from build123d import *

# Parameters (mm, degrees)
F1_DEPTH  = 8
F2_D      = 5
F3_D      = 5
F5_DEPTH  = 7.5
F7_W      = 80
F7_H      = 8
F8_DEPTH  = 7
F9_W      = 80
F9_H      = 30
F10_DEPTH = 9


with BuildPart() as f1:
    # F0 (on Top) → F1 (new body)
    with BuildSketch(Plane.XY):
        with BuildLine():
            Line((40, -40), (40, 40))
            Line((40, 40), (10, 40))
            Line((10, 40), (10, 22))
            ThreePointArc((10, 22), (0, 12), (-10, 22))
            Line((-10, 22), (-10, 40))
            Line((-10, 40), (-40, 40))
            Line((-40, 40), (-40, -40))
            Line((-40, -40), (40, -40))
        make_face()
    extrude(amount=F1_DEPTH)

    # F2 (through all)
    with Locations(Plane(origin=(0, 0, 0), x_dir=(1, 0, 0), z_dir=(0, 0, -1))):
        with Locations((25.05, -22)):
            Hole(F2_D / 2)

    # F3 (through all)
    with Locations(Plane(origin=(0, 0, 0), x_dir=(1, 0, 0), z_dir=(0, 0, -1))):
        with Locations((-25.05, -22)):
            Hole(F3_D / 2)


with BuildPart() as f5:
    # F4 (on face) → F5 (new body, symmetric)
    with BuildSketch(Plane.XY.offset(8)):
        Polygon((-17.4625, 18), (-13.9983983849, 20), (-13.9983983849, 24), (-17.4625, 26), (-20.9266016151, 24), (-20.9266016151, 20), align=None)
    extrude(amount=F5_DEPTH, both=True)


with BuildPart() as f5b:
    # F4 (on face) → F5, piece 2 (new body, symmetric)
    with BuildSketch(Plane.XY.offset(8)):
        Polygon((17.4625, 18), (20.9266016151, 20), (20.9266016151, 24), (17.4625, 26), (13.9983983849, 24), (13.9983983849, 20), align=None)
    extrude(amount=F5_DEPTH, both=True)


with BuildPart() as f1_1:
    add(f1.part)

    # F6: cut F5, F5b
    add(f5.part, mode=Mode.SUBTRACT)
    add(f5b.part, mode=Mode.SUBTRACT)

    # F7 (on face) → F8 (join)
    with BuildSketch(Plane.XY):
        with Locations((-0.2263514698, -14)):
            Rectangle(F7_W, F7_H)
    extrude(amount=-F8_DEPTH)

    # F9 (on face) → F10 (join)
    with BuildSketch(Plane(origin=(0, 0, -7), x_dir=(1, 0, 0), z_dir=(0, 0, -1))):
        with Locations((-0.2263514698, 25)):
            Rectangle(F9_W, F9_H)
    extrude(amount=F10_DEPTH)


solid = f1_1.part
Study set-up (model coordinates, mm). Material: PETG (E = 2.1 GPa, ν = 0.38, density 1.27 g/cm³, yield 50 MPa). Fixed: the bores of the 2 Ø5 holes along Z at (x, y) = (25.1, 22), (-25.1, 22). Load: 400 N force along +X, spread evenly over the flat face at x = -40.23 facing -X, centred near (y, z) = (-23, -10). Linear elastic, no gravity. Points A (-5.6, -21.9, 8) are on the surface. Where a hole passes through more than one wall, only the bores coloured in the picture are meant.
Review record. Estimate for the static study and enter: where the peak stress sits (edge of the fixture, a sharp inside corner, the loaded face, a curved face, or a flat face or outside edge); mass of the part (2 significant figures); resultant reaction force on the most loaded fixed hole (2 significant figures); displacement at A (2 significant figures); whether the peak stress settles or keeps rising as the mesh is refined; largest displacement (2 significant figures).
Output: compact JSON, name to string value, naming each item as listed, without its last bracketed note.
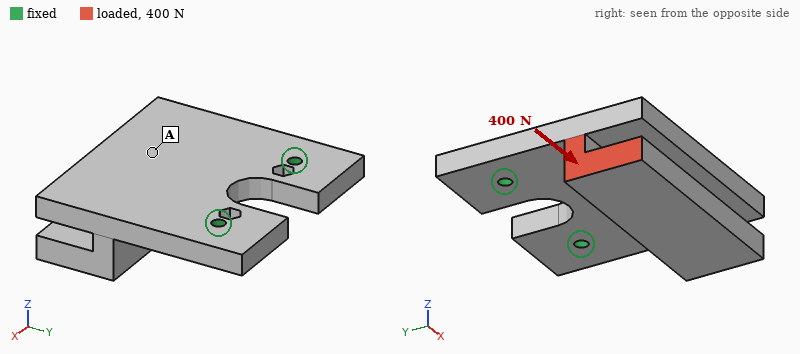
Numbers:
{"where the peak stress sits": "edge of the fixture", "mass of the part": "92 g", "resultant reaction force on the most loaded fixed hole": "390 N", "displacement at A": "0.058 mm", "whether the peak stress settles or keeps rising as the mesh is refined": "keeps rising", "largest displacement": "0.36 mm"}
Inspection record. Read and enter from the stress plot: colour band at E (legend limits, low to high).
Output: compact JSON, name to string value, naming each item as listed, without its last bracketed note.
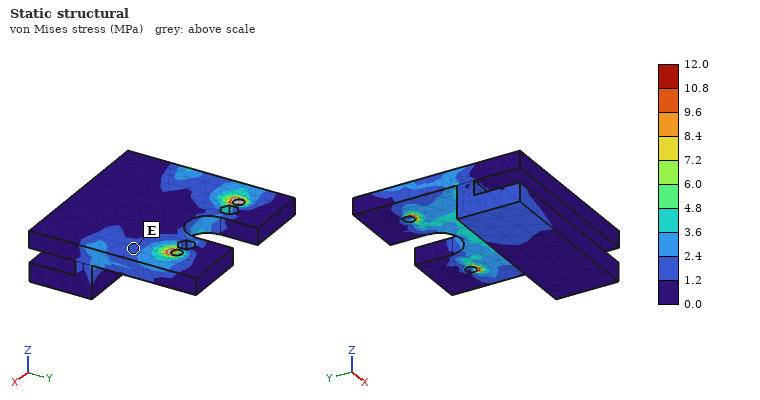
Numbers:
{"colour band at E": "1.2 to 2.4 MPa"}
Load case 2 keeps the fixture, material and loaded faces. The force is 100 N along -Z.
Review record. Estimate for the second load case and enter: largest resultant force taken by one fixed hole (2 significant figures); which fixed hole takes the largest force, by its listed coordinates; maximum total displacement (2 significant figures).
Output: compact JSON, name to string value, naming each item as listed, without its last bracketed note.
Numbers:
{"largest resultant force taken by one fixed hole": "120 N", "which fixed hole takes the largest force, by its listed coordinates": "(-25.1, 22)", "maximum total displacement": "1.3 mm"}
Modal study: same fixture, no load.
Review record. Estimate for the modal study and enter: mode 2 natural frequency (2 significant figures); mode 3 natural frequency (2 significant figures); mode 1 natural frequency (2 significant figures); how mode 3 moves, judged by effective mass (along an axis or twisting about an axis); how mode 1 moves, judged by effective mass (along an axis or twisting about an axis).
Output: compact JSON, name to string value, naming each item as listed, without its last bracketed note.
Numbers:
{"mode 2 natural frequency": "620 Hz", "mode 3 natural frequency": "1200 Hz", "mode 1 natural frequency": "240 Hz", "how mode 3 moves, judged by effective mass": "along X", "how mode 1 moves, judged by effective mass": "along Z"}
